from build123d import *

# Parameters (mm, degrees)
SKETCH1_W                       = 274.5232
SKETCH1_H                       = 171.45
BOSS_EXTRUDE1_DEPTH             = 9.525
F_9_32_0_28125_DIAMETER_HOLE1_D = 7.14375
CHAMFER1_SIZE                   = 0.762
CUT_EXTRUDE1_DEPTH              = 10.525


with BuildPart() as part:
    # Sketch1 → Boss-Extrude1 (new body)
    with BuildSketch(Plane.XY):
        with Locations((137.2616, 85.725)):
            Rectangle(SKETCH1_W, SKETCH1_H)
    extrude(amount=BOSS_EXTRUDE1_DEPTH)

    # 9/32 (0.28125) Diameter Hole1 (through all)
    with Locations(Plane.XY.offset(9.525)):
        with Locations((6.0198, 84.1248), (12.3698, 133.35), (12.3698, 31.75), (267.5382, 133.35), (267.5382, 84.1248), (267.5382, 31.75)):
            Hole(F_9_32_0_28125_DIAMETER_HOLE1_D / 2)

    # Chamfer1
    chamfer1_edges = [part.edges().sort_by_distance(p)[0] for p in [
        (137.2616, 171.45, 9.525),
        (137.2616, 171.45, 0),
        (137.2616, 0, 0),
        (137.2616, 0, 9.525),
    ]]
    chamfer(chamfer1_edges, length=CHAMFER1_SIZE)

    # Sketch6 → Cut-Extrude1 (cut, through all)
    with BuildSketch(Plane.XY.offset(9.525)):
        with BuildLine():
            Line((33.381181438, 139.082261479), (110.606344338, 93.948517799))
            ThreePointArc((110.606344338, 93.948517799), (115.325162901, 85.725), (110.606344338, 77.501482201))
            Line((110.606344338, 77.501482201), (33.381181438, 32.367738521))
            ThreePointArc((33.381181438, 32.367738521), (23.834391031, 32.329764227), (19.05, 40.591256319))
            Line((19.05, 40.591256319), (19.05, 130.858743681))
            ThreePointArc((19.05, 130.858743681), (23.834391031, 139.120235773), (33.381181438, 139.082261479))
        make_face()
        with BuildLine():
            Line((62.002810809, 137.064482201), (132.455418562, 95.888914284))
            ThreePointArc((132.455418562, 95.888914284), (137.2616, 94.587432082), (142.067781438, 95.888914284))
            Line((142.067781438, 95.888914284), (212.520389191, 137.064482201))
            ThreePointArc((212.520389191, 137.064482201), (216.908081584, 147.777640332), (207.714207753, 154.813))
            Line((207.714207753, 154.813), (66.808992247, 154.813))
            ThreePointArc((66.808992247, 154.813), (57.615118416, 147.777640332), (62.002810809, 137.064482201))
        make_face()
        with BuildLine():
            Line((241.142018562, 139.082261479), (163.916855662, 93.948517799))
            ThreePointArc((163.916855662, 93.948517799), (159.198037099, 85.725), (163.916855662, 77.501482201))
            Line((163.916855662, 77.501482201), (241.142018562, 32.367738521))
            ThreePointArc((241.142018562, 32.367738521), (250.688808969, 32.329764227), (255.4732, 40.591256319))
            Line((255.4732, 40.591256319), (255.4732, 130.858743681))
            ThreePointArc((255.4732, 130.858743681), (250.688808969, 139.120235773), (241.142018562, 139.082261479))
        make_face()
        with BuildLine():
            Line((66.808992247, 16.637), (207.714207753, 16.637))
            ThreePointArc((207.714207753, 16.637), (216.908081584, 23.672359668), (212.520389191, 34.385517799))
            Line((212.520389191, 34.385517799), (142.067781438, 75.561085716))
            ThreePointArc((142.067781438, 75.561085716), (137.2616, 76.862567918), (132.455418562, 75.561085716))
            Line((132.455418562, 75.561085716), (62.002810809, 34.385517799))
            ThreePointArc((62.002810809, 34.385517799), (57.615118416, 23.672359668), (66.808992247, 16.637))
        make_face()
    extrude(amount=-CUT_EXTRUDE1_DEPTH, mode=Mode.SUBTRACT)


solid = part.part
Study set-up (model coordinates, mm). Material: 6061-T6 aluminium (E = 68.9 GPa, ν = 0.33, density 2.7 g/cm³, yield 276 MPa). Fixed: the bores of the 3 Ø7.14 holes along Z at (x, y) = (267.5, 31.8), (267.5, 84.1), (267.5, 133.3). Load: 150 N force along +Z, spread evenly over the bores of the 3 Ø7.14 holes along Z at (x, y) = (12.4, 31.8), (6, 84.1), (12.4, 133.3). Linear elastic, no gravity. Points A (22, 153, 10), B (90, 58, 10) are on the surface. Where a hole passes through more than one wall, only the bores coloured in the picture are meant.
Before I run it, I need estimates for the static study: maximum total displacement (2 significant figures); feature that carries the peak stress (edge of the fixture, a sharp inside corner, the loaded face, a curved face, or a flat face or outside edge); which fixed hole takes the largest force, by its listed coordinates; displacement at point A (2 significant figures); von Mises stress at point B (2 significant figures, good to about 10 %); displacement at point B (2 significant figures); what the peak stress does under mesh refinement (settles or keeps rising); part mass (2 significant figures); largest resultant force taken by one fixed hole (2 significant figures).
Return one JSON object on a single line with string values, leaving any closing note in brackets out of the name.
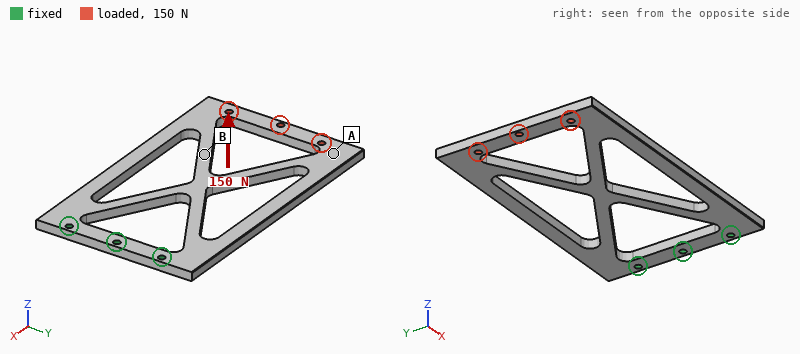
{"maximum total displacement": "3.3 mm", "feature that carries the peak stress": "edge of the fixture", "which fixed hole takes the largest force, by its listed coordinates": "(267.5, 31.8)", "displacement at point A": "2.9 mm", "von Mises stress at point B": "12 MPa", "displacement at point B": "1.7 mm", "what the peak stress does under mesh refinement": "keeps rising", "part mass": "560 g", "largest resultant force taken by one fixed hole": "120 N"}
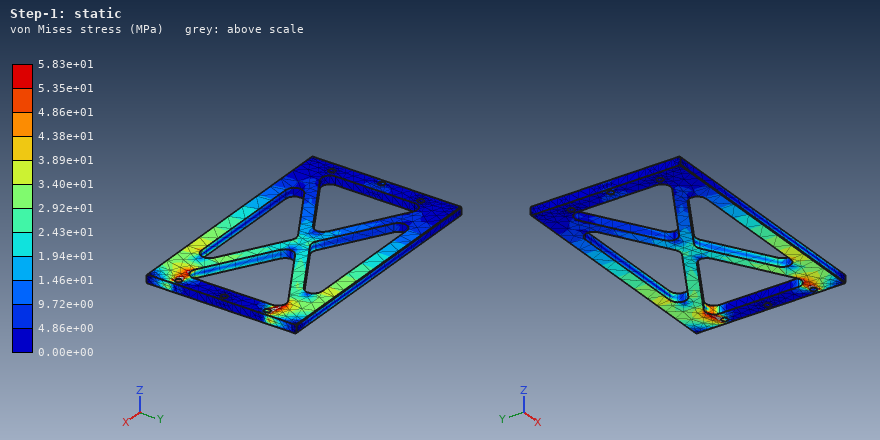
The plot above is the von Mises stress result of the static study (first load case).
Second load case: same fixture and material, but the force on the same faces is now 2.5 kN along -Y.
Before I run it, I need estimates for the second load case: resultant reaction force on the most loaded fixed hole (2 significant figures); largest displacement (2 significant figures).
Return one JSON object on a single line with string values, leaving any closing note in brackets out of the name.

{"resultant reaction force on the most loaded fixed hole": "5.2 kN", "largest displacement": "0.51 mm"}
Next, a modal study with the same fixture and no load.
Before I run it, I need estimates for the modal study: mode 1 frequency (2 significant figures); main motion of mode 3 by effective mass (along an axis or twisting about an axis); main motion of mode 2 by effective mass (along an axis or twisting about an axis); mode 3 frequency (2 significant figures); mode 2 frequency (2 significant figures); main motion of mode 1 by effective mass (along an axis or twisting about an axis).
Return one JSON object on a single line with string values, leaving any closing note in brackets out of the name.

{"mode 1 frequency": "83 Hz", "main motion of mode 3 by effective mass": "along Z", "main motion of mode 2 by effective mass": "twisting about X", "mode 3 frequency": "550 Hz", "mode 2 frequency": "240 Hz", "main motion of mode 1 by effective mass": "along Z"}
